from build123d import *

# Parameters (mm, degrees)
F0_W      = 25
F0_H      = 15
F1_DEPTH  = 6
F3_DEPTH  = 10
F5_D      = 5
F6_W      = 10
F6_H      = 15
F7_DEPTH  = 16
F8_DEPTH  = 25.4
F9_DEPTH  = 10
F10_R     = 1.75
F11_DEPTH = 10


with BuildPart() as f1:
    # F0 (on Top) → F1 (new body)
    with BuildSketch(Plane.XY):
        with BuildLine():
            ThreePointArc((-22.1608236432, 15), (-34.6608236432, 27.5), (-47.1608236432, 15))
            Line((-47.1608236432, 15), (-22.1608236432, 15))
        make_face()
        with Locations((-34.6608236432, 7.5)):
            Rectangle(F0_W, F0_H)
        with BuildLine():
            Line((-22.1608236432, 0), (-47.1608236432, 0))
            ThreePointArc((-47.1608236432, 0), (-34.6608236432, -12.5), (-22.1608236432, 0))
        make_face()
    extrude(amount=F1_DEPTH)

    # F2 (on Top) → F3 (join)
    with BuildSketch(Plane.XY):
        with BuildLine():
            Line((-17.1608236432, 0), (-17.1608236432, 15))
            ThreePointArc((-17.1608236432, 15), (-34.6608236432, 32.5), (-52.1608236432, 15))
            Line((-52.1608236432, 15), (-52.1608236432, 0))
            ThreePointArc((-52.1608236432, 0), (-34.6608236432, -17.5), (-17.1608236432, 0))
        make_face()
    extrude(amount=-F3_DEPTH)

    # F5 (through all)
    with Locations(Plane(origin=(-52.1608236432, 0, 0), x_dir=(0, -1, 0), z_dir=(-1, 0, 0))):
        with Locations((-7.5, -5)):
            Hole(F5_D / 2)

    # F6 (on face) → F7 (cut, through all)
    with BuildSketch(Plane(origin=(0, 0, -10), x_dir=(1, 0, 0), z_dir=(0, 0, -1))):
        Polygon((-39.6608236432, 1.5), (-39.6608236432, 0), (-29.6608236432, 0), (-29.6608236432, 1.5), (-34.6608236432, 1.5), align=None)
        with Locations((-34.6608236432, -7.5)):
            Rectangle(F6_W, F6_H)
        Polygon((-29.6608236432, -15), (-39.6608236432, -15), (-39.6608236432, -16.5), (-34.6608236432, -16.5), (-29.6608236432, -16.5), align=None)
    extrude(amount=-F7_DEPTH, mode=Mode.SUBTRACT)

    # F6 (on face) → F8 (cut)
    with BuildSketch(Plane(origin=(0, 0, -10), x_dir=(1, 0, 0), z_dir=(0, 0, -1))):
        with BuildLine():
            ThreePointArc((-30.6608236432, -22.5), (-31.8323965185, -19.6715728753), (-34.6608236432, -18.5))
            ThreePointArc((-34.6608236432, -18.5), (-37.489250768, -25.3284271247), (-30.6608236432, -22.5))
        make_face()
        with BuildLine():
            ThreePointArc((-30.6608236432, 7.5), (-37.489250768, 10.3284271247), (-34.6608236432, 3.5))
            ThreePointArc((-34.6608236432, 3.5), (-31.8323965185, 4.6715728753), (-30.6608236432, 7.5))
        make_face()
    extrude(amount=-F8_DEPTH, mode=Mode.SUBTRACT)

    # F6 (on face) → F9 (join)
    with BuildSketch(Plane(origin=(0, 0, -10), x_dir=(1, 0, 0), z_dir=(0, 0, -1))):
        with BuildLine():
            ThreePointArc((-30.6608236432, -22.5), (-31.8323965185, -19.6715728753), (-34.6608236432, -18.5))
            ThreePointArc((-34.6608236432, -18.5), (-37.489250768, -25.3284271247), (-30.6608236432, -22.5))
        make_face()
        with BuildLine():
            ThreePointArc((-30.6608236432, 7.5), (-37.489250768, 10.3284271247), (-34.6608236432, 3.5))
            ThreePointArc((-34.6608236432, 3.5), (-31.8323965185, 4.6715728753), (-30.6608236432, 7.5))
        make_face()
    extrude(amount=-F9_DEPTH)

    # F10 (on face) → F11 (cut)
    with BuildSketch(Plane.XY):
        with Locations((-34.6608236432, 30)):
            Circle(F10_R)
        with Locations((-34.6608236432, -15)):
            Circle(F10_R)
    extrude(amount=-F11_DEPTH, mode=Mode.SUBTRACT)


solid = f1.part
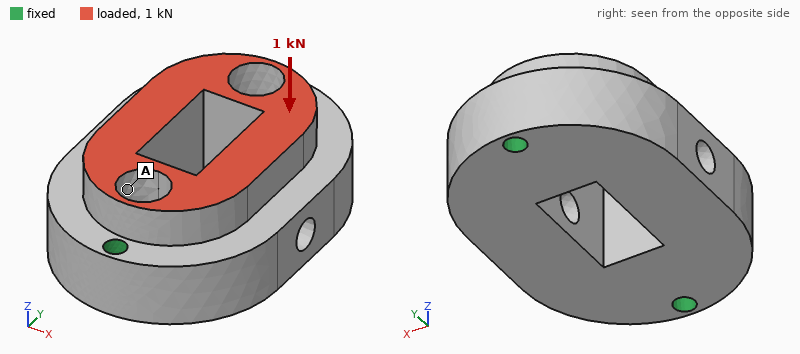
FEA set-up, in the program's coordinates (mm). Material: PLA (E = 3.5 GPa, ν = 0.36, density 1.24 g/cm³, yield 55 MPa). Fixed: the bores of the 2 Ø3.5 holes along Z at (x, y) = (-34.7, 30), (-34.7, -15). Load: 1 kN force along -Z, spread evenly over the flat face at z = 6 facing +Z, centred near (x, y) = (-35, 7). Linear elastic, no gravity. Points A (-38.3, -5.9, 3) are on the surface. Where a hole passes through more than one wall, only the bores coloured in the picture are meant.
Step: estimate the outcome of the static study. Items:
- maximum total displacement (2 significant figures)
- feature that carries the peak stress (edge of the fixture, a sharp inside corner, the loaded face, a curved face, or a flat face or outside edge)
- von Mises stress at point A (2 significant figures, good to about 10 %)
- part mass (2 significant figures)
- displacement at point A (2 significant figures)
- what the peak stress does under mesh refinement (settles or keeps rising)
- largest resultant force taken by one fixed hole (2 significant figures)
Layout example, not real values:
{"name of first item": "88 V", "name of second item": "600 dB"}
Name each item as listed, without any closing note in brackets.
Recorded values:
{"maximum total displacement": "71 µm", "feature that carries the peak stress": "edge of the fixture", "von Mises stress at point A": "3.5 MPa", "part mass": "20 g", "displacement at point A": "42 µm", "what the peak stress does under mesh refinement": "keeps rising", "largest resultant force taken by one fixed hole": "530 N"}
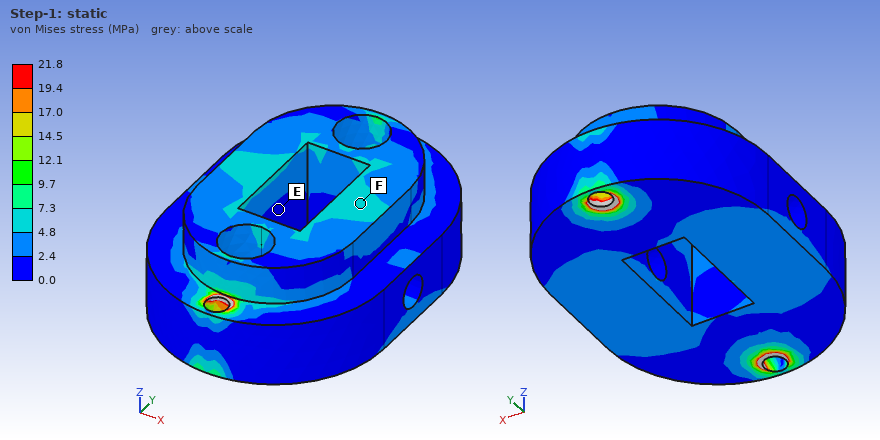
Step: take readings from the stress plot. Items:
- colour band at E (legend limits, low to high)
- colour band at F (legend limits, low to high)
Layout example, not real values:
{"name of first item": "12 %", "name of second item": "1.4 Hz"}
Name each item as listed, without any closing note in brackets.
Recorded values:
{"colour band at E": "0.0 to 2.4 MPa", "colour band at F": "4.8 to 7.3 MPa"}
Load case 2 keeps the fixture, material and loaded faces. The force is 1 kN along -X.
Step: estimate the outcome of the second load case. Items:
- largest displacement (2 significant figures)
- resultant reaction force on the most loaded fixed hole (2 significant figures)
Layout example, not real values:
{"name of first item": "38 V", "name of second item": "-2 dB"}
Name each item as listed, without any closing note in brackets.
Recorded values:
{"largest displacement": "0.21 mm", "resultant reaction force on the most loaded fixed hole": "500 N"}
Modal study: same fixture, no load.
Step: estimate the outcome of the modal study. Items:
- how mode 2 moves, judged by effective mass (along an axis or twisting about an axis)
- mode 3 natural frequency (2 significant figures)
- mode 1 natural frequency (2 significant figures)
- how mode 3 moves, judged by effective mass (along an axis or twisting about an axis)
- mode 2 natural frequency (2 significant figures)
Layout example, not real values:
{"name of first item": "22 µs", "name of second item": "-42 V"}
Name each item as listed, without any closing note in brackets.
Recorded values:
{"how mode 2 moves, judged by effective mass": "along Z", "mode 3 natural frequency": "7700 Hz", "mode 1 natural frequency": "3800 Hz", "how mode 3 moves, judged by effective mass": "along X", "mode 2 natural frequency": "5100 Hz"}
